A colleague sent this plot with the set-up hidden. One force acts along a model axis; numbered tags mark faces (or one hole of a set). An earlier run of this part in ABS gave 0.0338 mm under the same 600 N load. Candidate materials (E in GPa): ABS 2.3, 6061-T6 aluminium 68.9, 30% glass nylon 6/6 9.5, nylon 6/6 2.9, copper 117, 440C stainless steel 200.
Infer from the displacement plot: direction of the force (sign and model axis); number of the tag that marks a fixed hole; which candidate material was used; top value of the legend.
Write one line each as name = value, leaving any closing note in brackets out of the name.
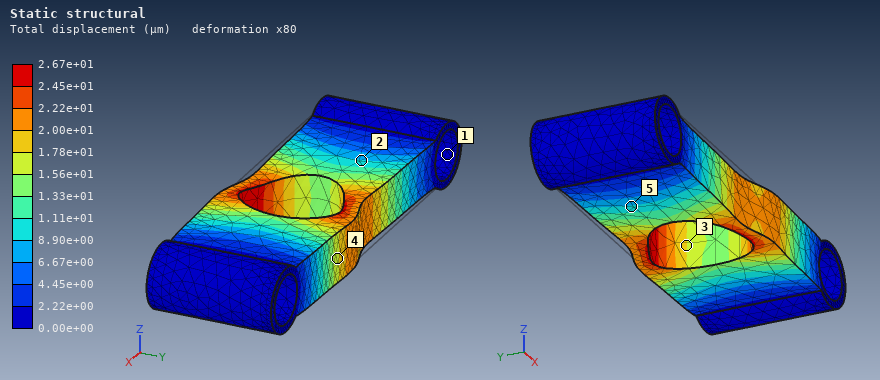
direction of the force = +X
number of the tag that marks a fixed hole = 1
which candidate material was used = nylon 6/6
top value of the legend = 2.67e+01 µm
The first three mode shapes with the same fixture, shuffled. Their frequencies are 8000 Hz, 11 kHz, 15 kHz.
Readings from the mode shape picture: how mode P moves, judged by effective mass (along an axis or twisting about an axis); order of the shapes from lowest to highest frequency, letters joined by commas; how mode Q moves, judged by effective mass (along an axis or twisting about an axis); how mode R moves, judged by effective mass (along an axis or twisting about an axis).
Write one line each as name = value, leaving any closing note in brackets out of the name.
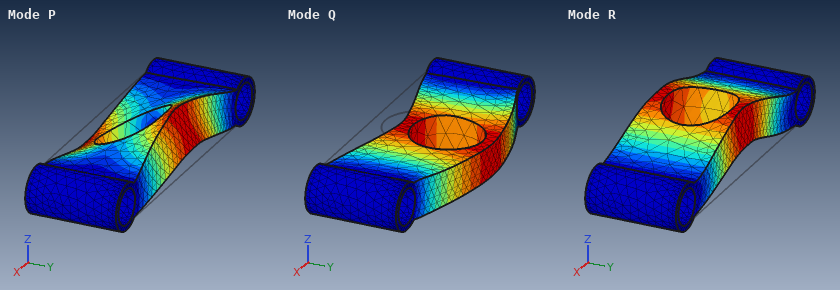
how mode P moves, judged by effective mass = twisting about X
order of the shapes from lowest to highest frequency, letters joined by commas = R, P, Q
how mode Q moves, judged by effective mass = along Y
how mode R moves, judged by effective mass = along Z
